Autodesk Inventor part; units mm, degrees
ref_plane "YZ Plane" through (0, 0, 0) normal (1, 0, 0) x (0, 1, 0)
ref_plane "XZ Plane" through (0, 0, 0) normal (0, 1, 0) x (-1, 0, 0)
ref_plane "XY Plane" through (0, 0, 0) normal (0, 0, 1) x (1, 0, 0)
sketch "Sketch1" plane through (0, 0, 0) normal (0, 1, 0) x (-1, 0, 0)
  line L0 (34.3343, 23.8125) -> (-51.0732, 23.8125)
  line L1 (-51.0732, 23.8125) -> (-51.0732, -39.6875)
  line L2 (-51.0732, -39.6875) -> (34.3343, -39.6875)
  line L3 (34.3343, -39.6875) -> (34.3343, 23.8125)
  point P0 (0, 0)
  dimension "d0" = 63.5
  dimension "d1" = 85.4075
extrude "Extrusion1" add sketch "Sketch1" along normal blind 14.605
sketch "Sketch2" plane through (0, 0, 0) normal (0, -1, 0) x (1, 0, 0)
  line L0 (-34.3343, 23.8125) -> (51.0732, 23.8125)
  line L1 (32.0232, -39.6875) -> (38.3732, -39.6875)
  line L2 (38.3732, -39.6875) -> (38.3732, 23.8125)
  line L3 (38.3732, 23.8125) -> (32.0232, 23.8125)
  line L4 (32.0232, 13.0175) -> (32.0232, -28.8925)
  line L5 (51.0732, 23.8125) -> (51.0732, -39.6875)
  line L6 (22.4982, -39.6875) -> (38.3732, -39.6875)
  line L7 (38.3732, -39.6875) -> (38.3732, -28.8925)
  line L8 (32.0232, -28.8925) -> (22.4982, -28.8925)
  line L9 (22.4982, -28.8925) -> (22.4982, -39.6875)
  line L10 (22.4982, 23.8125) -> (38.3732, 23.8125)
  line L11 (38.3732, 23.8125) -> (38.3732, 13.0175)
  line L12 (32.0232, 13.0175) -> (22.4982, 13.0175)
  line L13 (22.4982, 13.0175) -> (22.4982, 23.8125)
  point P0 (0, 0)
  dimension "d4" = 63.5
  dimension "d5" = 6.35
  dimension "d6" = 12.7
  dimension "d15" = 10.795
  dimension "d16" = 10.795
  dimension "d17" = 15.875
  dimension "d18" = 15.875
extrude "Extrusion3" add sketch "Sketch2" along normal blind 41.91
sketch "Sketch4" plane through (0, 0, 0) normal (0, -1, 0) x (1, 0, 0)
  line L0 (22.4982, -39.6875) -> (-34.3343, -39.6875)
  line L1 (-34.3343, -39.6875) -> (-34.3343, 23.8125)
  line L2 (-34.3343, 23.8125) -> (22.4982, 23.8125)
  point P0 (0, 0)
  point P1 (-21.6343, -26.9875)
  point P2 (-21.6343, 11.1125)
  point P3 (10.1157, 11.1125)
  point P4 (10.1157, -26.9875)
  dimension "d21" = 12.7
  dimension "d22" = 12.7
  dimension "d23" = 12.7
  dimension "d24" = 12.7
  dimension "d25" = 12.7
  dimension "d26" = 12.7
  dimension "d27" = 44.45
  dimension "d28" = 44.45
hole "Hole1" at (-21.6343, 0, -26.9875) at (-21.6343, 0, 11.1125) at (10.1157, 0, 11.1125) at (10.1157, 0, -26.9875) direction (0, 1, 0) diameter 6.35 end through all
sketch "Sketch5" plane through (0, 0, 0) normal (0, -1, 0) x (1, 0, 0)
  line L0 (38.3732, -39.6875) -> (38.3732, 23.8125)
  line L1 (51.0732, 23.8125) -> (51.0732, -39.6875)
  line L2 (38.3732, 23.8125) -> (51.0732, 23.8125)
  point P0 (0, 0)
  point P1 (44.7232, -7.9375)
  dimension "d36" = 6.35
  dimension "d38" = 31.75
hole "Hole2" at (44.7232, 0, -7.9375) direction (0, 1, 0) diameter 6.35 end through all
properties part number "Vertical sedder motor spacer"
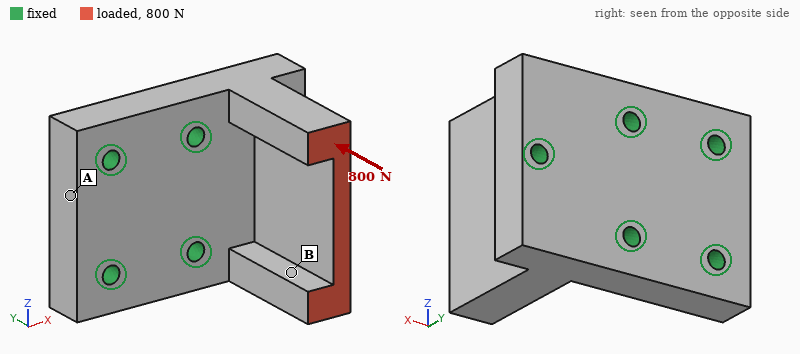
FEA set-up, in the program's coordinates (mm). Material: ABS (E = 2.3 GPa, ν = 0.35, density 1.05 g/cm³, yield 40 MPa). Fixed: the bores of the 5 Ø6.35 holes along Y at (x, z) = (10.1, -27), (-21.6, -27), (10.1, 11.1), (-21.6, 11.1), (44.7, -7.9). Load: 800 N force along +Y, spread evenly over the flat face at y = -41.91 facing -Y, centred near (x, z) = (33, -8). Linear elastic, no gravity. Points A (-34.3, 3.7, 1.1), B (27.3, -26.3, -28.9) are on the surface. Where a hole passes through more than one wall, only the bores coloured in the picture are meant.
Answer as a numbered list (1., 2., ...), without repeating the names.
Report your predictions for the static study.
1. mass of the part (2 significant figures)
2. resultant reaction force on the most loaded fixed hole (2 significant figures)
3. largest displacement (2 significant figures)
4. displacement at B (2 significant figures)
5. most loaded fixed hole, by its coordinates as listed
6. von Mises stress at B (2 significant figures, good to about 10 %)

1. 110 g
2. 450 N
3. 52 µm
4. 41 µm
5. (44.7, -7.9)
6. 1.4 MPa
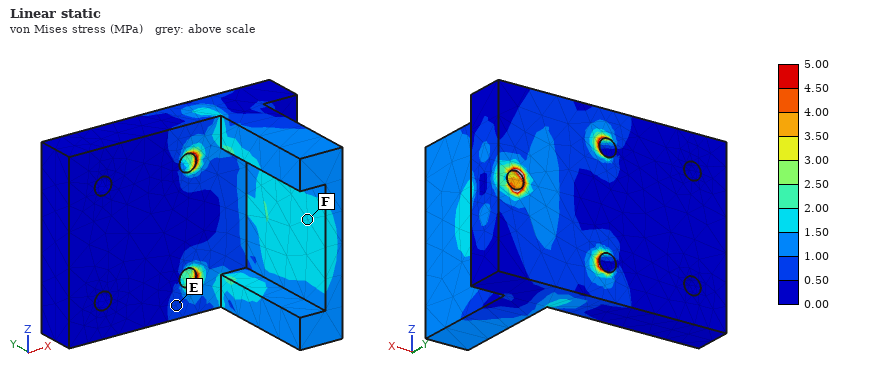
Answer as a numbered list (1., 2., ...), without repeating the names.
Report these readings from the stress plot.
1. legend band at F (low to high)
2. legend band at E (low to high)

1. 1.50 to 2.00 MPa
2. 0.50 to 1.00 MPa
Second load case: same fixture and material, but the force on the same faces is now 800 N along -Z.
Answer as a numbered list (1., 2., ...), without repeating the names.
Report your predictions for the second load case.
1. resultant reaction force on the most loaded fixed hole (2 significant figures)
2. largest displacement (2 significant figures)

1. 610 N
2. 0.69 mm
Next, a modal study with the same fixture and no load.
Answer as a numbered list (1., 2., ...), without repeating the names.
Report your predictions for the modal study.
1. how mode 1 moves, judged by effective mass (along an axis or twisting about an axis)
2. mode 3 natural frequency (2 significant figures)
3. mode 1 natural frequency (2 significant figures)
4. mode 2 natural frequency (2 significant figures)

1. along X
2. 2300 Hz
3. 1400 Hz
4. 1500 Hz
